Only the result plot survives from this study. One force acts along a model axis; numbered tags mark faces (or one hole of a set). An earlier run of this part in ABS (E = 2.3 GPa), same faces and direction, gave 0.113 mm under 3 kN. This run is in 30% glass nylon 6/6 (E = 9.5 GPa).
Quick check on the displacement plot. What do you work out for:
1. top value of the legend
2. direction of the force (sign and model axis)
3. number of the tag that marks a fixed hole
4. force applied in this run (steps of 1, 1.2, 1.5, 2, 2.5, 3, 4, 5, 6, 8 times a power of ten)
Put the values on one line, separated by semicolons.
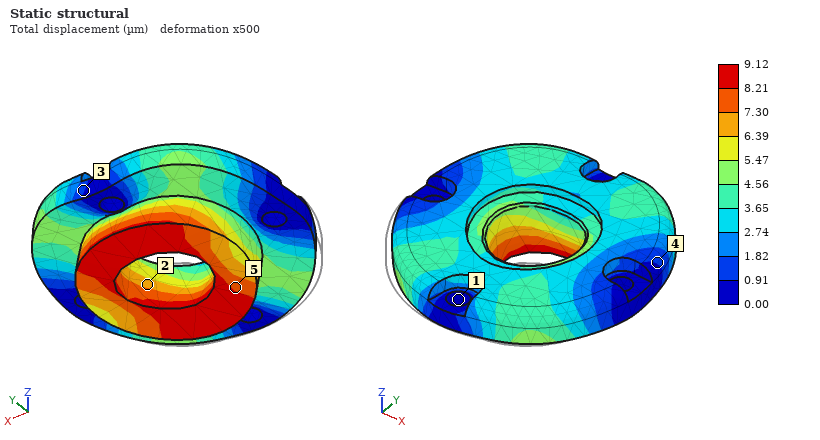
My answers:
9.12 µm; +Y; 1; 1 kN
